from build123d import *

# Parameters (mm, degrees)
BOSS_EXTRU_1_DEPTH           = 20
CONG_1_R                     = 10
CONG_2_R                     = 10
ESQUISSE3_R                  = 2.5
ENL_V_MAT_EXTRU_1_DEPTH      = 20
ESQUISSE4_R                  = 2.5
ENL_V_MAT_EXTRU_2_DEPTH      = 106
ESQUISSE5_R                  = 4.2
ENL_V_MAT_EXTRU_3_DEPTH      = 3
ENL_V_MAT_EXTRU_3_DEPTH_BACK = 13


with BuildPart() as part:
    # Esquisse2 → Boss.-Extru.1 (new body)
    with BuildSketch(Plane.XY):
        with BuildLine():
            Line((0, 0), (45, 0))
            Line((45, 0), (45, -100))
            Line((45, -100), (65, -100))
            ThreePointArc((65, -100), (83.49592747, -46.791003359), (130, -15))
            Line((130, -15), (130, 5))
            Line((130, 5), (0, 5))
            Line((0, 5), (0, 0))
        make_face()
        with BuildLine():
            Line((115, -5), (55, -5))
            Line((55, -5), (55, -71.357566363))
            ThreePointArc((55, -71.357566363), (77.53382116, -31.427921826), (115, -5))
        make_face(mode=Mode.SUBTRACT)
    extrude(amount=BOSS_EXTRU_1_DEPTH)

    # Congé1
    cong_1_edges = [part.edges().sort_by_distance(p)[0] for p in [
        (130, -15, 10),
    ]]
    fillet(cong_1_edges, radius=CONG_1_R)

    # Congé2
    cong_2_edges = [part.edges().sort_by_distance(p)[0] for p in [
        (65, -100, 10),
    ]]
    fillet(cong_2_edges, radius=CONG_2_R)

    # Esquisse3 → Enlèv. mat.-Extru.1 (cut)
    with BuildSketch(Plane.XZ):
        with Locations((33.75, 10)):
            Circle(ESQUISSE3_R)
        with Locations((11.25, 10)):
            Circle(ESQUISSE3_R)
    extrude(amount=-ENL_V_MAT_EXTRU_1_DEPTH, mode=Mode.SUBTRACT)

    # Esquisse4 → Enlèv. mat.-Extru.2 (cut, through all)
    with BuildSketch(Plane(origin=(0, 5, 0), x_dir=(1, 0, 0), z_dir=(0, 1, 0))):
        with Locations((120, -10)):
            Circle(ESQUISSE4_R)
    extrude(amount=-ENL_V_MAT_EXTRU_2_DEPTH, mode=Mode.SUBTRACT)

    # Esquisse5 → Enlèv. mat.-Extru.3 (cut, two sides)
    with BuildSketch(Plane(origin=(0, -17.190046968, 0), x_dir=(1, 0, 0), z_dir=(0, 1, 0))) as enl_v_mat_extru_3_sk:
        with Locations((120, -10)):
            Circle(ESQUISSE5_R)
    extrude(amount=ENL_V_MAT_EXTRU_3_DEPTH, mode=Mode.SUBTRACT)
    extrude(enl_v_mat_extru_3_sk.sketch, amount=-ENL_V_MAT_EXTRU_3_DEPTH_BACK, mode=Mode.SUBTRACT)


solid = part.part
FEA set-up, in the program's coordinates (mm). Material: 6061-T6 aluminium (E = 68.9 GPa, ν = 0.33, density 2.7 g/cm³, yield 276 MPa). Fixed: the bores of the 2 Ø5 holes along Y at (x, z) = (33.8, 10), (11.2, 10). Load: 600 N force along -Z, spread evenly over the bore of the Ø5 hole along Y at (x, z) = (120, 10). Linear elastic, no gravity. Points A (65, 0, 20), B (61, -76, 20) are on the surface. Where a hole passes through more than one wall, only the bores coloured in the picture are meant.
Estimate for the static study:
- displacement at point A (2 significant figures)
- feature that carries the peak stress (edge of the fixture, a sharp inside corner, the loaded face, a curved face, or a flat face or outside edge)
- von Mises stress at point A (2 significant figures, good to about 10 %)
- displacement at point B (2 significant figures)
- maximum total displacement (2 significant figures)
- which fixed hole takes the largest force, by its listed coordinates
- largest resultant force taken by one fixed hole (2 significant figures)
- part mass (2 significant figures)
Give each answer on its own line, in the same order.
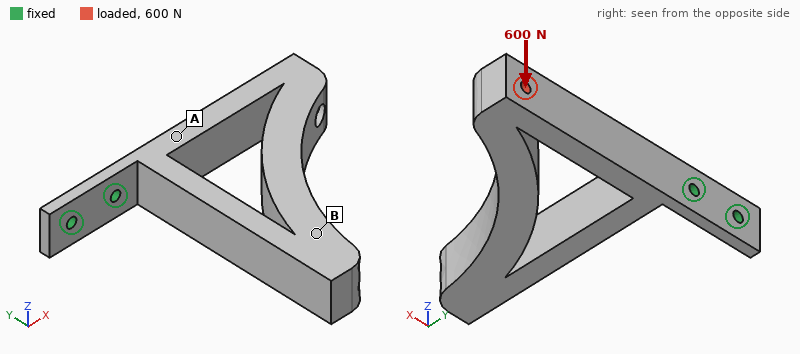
0.16 mm
edge of the fixture
46 MPa
0.24 mm
0.65 mm
(33.8, 10)
2.0 kN
200 g
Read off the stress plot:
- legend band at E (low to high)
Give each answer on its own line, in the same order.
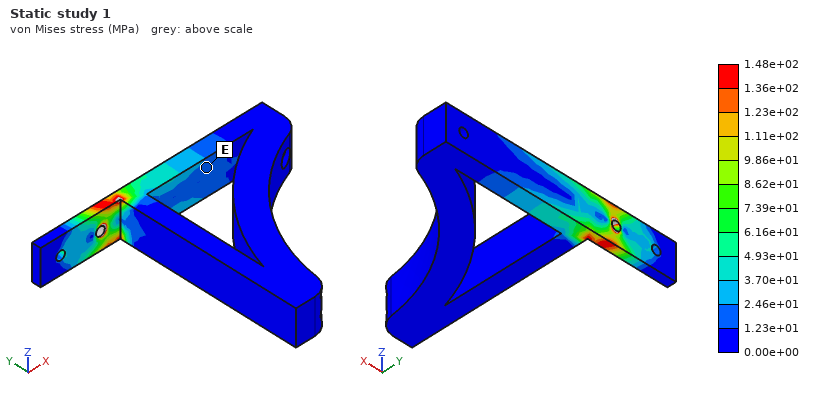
1.23e+01 to 2.46e+01 MPa
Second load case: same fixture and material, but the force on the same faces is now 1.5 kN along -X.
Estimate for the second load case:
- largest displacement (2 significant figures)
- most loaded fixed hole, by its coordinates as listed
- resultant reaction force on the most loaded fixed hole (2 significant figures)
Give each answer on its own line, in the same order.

1.0 mm
(33.8, 10)
1.3 kN
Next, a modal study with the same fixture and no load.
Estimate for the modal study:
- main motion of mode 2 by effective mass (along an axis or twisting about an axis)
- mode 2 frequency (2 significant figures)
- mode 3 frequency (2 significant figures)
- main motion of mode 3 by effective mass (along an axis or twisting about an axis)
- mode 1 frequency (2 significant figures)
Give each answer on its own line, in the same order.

along Z
320 Hz
800 Hz
along Z
190 Hz
